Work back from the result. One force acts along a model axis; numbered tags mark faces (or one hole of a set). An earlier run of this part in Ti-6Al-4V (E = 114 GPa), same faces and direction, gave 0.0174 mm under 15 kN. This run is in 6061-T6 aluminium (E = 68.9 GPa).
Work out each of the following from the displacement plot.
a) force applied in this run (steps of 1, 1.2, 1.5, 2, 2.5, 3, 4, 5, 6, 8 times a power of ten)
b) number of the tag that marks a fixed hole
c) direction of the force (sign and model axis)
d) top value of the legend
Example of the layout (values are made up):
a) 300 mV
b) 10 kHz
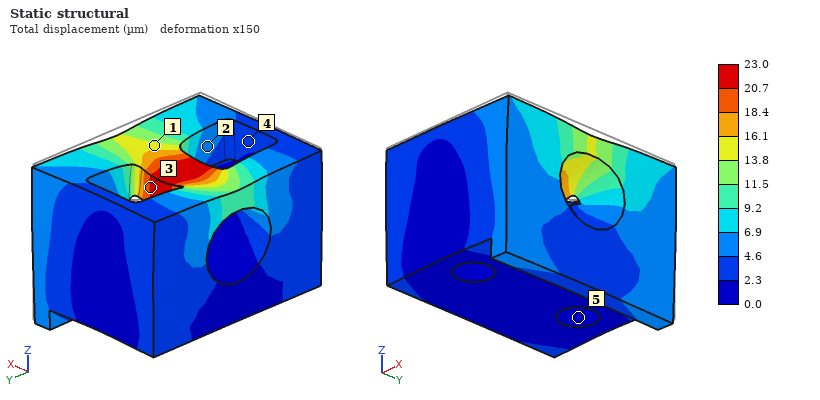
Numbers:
a) 12 kN
b) 5
c) -Z
d) 23.0 µm
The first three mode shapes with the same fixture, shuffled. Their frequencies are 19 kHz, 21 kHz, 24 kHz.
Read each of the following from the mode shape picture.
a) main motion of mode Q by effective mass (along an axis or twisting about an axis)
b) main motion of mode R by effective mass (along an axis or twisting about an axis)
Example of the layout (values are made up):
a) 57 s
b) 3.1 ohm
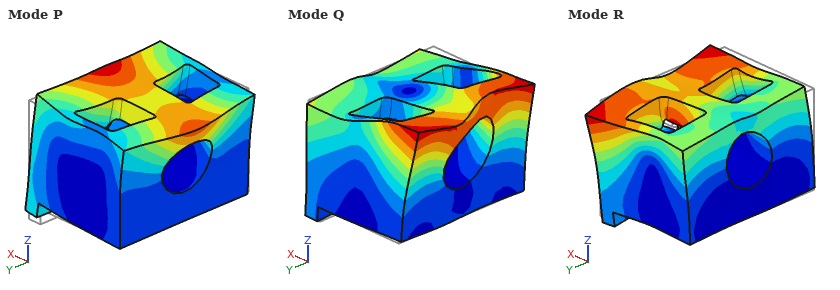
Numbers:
a) twisting about Z
b) along Y
